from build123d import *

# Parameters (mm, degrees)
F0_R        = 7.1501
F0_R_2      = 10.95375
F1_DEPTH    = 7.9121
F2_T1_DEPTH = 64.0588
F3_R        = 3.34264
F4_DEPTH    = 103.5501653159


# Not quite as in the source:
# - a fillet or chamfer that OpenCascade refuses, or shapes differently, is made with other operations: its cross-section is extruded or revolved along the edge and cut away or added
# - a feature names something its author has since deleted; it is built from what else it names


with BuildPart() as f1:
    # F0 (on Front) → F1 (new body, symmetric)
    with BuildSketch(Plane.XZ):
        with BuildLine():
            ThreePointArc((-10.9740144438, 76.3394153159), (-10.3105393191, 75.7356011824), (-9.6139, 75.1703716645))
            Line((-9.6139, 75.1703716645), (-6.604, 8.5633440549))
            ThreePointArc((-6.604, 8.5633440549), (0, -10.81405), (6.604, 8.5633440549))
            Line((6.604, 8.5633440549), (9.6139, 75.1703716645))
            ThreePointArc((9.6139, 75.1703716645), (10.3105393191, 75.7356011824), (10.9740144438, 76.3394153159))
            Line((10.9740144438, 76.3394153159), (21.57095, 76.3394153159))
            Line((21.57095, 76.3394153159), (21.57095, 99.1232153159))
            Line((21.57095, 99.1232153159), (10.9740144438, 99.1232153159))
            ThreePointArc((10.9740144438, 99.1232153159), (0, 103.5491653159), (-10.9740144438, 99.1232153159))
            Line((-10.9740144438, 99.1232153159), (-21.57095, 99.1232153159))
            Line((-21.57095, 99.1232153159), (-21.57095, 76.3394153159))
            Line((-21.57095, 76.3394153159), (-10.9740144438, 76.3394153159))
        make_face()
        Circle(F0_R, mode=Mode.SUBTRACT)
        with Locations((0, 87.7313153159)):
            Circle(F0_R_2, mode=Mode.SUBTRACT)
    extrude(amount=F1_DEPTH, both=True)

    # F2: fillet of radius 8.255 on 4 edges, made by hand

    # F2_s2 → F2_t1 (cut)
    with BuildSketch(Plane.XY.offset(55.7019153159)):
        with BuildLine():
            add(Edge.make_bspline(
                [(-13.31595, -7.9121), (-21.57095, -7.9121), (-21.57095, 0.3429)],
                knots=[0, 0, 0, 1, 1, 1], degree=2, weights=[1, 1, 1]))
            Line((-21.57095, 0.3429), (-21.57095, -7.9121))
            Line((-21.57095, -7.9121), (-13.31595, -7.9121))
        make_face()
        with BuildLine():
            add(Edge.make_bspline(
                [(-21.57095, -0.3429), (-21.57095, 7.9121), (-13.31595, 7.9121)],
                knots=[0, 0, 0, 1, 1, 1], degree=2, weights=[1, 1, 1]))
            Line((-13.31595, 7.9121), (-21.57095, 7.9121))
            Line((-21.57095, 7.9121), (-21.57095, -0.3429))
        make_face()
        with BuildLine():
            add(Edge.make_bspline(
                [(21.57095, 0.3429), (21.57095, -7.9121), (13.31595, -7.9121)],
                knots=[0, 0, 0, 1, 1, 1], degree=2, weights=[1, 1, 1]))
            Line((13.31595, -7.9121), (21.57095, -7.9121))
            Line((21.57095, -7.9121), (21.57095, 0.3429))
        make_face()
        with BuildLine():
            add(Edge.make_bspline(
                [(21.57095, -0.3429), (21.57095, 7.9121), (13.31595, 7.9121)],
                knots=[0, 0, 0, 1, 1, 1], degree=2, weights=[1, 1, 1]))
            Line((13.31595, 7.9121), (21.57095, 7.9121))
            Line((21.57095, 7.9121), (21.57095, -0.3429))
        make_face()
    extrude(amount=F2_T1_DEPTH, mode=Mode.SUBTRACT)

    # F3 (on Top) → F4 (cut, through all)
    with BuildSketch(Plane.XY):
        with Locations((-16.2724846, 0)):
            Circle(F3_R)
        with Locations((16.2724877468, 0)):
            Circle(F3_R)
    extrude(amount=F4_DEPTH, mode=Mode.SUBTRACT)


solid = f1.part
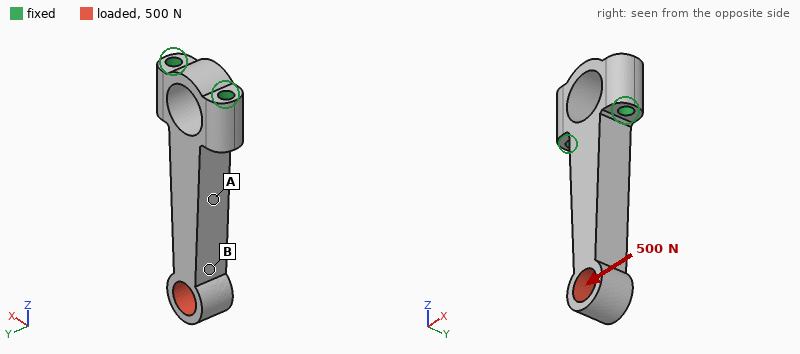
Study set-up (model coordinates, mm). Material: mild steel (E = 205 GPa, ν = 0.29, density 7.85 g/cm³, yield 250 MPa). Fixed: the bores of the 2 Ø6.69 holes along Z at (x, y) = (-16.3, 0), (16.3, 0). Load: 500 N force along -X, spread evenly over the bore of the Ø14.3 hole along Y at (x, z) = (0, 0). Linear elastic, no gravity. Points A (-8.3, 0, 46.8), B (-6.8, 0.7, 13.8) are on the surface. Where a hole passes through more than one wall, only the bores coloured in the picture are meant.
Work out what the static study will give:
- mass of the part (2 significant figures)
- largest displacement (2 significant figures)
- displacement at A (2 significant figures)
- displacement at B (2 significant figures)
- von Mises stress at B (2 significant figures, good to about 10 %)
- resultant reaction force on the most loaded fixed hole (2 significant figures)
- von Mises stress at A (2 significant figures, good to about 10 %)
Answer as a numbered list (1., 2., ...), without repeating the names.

1. 220 g
2. 93 µm
3. 17 µm
4. 54 µm
5. 15 MPa
6. 2.0 kN
7. 32 MPa
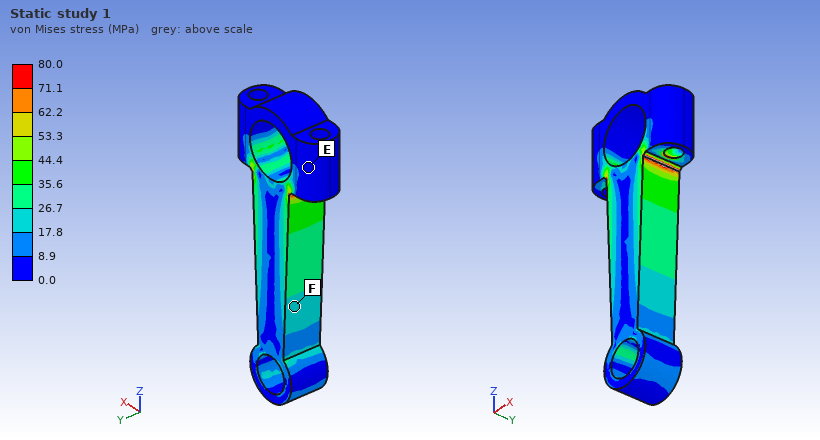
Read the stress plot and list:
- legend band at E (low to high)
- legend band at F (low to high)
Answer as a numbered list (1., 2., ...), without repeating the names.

1. 0.0 to 8.9 MPa
2. 17.8 to 26.7 MPa
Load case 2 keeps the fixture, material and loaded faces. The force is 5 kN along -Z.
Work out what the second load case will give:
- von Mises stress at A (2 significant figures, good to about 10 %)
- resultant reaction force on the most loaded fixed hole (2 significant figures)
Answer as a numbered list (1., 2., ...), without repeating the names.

1. 19 MPa
2. 2.9 kN
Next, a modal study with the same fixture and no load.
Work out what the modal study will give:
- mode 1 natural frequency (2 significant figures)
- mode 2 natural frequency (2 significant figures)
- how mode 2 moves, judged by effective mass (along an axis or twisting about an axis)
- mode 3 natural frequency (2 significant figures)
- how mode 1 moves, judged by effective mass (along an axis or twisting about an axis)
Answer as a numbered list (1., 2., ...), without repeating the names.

1. 1300 Hz
2. 1900 Hz
3. along X
4. 7600 Hz
5. along Y
